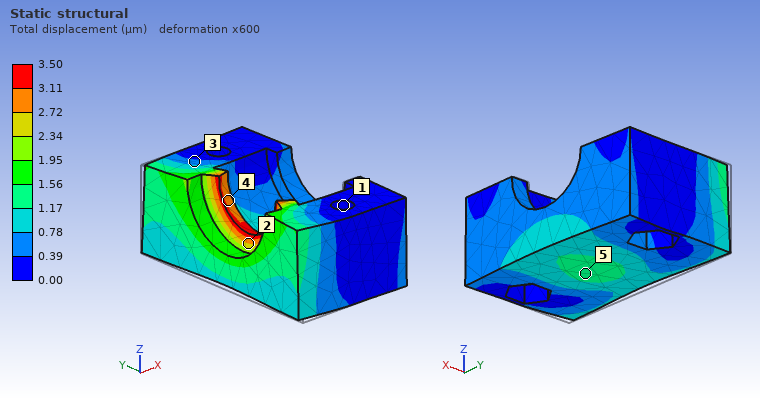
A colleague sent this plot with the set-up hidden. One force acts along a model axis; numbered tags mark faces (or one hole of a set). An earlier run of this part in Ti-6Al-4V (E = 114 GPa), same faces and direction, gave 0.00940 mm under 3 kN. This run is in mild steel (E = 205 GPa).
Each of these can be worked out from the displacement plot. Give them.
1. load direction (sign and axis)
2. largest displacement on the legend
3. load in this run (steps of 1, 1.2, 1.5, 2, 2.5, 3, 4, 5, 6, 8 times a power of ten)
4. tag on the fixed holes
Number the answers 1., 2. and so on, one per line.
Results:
1. +X
2. 3.50 µm
3. 2 kN
4. 1
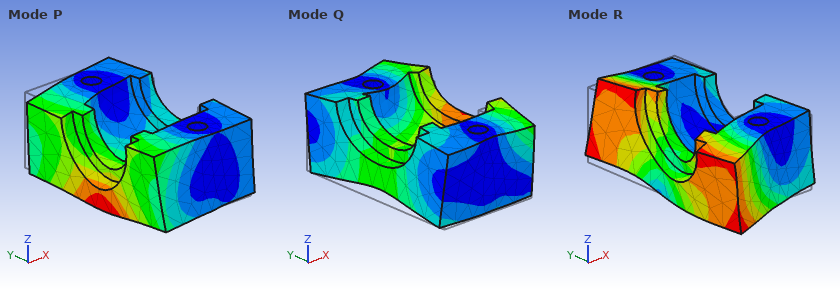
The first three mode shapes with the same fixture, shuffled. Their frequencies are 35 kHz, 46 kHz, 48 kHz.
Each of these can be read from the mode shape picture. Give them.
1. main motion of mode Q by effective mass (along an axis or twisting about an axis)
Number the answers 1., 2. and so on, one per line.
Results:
1. along Z
